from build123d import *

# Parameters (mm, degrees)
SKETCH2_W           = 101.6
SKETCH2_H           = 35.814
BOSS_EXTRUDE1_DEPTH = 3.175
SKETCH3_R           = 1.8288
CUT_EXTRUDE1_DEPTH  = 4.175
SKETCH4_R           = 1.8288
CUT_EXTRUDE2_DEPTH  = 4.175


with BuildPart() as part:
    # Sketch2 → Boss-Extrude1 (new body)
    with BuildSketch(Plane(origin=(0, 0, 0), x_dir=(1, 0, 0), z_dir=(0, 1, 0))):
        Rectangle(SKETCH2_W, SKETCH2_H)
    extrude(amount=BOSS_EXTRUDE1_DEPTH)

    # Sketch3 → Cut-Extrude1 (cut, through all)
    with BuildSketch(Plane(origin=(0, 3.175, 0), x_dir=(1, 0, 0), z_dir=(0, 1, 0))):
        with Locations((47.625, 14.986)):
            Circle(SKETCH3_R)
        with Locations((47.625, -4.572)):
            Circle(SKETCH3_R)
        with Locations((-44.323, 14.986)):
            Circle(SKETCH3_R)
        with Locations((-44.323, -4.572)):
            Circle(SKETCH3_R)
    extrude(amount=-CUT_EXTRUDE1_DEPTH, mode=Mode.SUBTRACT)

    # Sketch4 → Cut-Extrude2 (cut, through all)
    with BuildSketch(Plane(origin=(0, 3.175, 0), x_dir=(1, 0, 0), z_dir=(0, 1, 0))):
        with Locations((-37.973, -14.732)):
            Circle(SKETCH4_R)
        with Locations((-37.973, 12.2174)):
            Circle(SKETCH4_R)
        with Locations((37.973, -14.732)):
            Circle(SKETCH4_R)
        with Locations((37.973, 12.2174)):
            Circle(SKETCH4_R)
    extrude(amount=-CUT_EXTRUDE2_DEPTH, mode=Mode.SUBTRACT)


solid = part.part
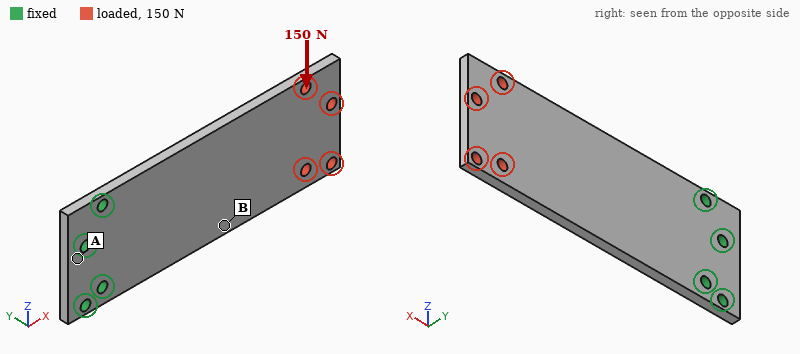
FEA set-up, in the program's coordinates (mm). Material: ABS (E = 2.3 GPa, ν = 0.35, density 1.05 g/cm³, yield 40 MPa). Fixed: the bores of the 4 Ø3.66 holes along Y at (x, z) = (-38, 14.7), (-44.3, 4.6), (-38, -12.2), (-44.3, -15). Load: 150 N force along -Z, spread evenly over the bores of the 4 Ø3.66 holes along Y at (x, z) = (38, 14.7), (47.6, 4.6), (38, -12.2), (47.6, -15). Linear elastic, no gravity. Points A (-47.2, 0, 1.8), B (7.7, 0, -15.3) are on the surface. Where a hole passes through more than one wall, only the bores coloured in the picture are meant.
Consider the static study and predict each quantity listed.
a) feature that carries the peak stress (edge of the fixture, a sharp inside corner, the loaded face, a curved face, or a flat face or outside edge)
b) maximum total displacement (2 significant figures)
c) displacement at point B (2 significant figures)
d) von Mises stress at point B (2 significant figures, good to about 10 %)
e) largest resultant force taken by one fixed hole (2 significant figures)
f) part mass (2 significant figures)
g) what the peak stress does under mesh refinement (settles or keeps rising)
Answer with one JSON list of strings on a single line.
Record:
["edge of the fixture", "1.3 mm", "0.51 mm", "6.7 MPa", "400 N", "12 g", "keeps rising"]
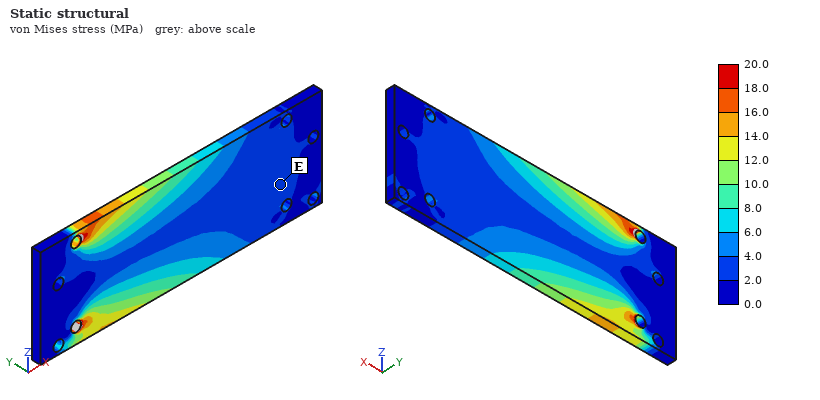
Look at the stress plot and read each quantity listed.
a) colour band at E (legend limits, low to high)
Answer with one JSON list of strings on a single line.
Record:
["2.0 to 4.0 MPa"]
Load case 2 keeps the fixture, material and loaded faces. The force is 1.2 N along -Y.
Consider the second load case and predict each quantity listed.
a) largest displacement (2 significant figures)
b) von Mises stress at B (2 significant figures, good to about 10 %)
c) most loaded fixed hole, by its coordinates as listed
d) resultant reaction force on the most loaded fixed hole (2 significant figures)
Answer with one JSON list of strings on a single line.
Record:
["1.1 mm", "0.72 MPa", "(-38, -12.2)", "3.3 N"]
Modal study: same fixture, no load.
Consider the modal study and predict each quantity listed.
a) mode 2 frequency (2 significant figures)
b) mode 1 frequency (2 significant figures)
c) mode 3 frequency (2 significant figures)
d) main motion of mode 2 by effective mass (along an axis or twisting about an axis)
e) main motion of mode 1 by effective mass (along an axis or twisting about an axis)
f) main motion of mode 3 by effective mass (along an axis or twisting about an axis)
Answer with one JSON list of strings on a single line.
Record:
["500 Hz", "99 Hz", "610 Hz", "twisting about X", "along Y", "along Y"]
